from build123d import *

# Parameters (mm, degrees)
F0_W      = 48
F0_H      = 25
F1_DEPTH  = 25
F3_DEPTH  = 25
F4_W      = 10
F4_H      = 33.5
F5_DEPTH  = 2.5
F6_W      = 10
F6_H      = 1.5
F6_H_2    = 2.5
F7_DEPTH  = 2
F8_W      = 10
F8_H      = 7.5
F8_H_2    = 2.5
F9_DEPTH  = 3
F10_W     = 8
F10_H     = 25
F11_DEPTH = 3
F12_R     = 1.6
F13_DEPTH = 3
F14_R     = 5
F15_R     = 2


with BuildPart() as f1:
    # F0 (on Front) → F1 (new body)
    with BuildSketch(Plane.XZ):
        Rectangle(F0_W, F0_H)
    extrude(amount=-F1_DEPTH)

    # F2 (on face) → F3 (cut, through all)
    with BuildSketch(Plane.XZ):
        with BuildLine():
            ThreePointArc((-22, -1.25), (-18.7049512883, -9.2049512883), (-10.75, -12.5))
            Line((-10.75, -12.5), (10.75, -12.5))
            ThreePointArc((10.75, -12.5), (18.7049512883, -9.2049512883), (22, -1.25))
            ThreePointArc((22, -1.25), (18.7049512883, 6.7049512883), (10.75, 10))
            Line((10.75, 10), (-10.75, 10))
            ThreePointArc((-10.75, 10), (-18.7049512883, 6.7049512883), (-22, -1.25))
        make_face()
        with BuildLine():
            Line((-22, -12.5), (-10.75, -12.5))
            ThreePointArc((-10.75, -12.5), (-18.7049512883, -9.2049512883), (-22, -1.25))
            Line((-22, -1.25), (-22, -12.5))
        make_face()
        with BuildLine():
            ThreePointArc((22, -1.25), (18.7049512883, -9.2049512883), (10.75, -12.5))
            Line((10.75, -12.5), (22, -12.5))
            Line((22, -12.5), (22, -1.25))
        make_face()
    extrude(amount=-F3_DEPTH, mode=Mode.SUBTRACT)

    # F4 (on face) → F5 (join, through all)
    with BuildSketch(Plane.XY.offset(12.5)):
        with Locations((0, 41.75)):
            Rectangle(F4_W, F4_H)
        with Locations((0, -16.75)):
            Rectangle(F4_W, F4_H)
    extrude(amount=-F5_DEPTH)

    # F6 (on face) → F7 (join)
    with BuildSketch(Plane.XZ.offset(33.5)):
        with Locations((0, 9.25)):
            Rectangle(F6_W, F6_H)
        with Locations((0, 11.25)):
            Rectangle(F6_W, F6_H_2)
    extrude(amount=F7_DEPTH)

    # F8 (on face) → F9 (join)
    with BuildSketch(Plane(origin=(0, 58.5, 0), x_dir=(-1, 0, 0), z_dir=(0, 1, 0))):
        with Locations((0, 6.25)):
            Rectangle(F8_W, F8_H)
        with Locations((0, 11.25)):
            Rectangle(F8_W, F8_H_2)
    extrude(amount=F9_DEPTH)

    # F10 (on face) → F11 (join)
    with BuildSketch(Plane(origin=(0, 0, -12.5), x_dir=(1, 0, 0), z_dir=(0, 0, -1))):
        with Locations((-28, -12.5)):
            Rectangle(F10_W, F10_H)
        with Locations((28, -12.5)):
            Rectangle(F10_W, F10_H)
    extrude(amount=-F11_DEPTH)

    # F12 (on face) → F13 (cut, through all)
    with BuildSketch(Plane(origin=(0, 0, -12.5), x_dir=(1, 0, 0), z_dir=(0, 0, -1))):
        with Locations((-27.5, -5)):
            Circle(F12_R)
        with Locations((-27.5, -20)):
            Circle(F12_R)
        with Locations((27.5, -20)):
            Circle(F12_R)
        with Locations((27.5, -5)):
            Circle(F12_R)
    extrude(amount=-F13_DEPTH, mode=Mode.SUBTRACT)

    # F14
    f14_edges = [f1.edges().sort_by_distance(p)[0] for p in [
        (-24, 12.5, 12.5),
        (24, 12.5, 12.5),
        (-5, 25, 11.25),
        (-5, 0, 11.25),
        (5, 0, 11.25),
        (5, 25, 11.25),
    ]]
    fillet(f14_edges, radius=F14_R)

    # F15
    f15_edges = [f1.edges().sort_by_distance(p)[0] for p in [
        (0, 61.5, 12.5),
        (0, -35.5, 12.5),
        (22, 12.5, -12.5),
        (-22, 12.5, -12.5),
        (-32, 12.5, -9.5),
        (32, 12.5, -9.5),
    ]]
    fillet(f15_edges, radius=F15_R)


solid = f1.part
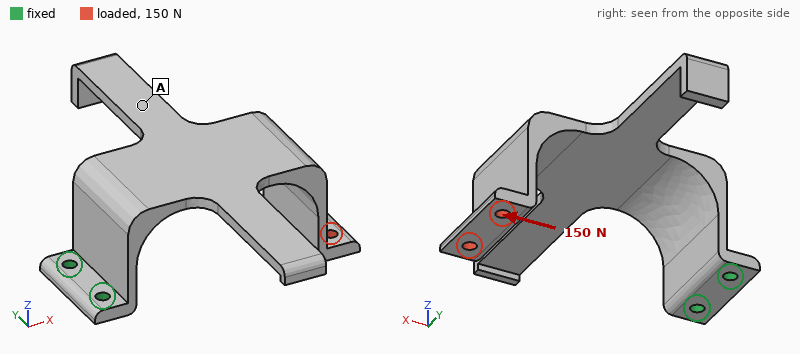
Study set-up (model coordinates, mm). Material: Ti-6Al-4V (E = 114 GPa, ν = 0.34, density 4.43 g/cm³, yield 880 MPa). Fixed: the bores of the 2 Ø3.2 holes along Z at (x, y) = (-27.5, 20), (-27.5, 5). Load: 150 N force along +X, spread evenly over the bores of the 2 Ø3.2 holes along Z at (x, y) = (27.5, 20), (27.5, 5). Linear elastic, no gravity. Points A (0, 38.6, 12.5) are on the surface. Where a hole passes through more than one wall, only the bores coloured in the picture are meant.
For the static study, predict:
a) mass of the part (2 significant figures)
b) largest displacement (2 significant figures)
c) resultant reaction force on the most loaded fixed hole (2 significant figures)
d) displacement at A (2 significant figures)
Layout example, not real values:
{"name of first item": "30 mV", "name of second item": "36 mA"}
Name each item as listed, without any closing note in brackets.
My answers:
{"mass of the part": "42 g", "largest displacement": "1.4 mm", "resultant reaction force on the most loaded fixed hole": "76 N", "displacement at A": "0.25 mm"}
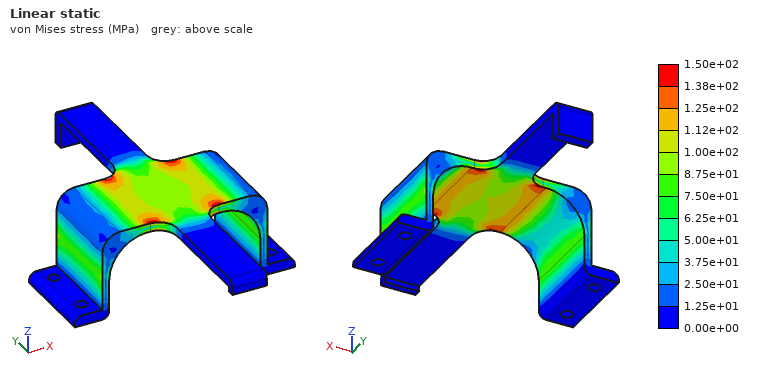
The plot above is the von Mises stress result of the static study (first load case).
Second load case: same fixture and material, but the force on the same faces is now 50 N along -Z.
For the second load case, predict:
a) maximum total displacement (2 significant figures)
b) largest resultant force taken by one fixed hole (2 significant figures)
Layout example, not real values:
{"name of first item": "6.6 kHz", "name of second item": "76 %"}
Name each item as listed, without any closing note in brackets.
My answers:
{"maximum total displacement": "1.4 mm", "largest resultant force taken by one fixed hole": "25 N"}
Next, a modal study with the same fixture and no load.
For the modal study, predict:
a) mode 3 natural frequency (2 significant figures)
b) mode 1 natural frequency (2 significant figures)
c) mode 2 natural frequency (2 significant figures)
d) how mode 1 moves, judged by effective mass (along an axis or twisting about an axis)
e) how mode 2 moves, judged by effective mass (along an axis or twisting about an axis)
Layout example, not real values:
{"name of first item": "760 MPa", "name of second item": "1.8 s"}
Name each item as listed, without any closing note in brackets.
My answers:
{"mode 3 natural frequency": "800 Hz", "mode 1 natural frequency": "270 Hz", "mode 2 natural frequency": "490 Hz", "how mode 1 moves, judged by effective mass": "along Z", "how mode 2 moves, judged by effective mass": "along Y"}
